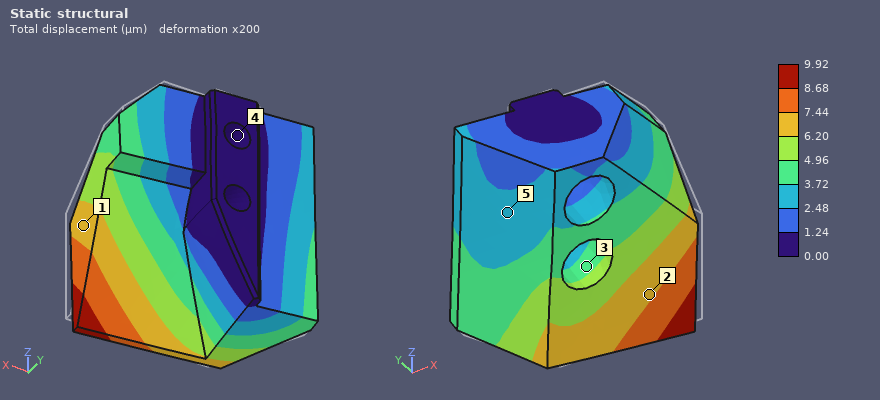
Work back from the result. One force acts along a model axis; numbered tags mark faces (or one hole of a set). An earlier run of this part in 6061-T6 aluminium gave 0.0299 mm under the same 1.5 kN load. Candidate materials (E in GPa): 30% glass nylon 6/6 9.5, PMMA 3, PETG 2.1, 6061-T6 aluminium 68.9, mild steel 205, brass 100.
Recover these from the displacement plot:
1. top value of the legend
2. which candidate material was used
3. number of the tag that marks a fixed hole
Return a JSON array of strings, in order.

["9.92 µm", "mild steel", "4"]
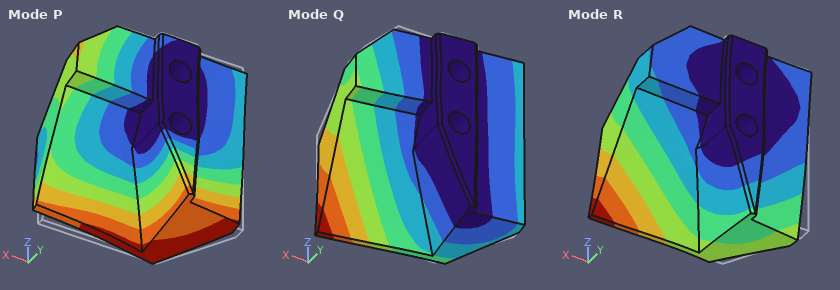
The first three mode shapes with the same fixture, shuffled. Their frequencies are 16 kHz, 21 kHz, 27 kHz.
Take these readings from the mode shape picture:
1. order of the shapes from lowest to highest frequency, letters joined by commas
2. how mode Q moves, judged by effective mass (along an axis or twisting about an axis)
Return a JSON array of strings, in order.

["Q, R, P", "along X"]
